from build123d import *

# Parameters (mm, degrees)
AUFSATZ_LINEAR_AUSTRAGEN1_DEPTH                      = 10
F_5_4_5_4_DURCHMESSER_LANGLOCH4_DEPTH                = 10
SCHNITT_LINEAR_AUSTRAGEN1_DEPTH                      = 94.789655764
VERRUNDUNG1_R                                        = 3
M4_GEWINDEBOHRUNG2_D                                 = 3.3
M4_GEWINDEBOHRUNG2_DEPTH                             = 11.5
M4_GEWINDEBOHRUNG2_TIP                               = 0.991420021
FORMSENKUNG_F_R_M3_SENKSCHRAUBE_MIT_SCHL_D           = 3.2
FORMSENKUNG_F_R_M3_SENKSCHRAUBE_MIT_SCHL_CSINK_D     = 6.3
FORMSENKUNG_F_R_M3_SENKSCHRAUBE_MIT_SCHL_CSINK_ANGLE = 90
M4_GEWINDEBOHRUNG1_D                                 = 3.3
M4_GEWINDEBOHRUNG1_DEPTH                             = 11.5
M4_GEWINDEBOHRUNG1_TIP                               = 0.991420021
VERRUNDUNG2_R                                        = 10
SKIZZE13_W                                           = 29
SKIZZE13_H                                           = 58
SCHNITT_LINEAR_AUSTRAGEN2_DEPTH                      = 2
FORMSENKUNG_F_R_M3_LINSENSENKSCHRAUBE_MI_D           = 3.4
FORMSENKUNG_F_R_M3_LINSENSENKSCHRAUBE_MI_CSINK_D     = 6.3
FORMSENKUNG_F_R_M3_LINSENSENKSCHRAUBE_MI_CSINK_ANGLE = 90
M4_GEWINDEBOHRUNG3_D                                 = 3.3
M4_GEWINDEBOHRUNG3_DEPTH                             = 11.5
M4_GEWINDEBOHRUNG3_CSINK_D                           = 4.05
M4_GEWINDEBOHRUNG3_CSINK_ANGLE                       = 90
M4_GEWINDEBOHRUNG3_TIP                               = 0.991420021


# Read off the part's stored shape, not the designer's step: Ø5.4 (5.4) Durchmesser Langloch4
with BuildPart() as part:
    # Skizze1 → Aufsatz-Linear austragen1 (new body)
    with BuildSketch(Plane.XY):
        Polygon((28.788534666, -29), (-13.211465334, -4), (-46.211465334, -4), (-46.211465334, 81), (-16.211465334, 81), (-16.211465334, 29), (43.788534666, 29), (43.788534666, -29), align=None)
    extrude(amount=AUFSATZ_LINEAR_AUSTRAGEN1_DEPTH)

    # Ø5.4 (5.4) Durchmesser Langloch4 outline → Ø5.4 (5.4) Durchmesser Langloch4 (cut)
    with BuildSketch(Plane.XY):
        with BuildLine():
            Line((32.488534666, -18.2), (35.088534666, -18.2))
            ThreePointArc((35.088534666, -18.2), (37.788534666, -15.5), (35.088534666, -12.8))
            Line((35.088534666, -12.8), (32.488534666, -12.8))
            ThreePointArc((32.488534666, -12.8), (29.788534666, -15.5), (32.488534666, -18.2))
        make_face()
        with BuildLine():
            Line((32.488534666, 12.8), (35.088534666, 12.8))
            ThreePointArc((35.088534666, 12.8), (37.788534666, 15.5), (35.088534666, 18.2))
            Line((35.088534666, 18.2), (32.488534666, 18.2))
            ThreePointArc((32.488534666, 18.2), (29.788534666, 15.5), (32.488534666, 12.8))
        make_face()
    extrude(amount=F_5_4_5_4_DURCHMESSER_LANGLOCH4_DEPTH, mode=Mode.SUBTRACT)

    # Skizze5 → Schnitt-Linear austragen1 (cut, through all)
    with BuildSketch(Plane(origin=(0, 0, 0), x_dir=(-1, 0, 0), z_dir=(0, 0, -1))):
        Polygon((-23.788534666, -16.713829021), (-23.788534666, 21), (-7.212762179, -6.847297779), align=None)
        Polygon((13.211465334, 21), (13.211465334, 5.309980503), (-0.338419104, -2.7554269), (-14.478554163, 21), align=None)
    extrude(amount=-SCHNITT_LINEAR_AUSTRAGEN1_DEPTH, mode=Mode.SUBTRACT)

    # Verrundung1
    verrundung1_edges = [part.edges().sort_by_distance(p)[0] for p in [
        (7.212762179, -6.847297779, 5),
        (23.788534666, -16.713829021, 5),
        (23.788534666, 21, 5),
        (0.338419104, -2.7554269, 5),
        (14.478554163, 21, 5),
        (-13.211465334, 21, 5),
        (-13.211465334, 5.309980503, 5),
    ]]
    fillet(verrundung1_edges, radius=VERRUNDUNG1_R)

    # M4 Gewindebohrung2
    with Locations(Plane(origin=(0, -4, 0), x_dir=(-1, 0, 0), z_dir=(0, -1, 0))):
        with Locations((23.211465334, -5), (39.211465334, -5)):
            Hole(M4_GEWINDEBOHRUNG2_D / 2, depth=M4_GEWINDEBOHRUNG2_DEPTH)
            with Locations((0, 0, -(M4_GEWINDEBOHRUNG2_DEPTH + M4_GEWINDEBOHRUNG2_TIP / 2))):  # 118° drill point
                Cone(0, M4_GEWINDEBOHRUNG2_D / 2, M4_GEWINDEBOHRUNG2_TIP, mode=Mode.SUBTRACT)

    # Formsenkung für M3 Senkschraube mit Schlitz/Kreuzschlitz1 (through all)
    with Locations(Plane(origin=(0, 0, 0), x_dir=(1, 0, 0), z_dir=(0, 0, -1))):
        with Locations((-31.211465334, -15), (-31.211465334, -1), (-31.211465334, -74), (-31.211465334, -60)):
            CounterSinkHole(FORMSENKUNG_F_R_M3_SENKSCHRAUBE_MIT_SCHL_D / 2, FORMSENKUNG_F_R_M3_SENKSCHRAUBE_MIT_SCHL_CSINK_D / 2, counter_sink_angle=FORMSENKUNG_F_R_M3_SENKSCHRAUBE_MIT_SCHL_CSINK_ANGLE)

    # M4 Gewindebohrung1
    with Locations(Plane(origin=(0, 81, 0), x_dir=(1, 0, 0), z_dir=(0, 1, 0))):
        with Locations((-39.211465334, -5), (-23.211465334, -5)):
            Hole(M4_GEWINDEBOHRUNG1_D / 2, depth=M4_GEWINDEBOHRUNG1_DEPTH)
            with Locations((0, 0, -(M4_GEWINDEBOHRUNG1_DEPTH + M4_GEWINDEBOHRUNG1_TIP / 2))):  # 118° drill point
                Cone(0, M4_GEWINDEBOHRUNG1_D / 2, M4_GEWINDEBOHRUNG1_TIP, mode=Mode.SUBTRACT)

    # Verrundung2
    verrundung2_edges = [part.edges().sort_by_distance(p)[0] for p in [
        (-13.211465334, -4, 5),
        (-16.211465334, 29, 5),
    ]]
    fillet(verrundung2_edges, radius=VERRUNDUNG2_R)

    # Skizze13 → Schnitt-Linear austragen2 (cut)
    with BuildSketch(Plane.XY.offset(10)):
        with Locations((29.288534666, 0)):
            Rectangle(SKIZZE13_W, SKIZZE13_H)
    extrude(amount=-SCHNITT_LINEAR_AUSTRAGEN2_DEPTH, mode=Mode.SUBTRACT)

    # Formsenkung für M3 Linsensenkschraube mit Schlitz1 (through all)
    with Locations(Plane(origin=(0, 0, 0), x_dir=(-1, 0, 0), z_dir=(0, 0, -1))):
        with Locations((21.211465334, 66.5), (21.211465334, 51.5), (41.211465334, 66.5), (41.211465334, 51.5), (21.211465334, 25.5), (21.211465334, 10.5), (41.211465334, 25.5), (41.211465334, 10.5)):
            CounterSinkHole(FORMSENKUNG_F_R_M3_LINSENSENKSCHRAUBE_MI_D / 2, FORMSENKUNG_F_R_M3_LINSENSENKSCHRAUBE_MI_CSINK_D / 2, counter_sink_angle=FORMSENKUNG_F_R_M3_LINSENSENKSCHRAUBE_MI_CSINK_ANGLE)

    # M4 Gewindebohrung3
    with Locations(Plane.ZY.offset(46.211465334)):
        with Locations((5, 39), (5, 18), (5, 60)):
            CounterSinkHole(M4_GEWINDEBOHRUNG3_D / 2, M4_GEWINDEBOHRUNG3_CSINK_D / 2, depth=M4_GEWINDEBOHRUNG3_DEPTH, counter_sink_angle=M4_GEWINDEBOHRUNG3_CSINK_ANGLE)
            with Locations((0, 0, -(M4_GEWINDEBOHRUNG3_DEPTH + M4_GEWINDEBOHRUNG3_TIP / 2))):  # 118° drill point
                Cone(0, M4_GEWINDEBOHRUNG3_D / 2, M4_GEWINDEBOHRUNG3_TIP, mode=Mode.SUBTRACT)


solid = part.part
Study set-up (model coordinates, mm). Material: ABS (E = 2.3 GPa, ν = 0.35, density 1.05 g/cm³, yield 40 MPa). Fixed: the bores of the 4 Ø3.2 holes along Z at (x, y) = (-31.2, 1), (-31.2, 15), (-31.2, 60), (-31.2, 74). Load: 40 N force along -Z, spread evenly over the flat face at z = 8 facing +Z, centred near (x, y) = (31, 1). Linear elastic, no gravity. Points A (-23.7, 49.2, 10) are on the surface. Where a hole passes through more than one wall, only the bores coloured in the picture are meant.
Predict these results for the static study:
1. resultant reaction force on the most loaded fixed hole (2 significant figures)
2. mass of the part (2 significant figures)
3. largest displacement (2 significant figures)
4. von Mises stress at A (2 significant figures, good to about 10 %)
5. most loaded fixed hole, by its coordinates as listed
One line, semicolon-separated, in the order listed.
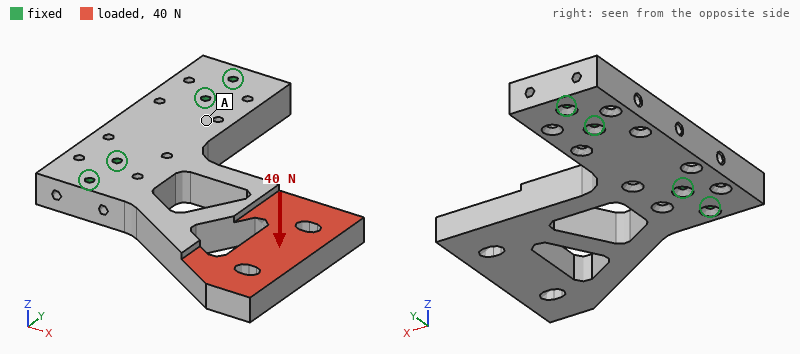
26 N; 44 g; 1.2 mm; 0.83 MPa; (-31.2, 15)
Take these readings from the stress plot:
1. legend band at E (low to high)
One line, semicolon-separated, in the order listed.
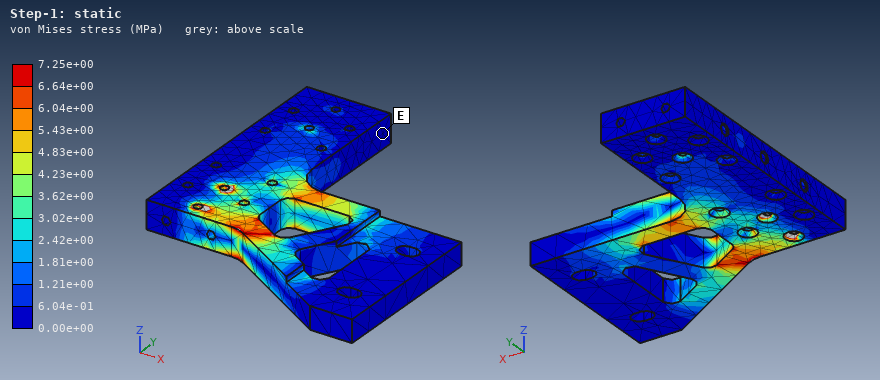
0.00e+00 to 6.04e-01 MPa
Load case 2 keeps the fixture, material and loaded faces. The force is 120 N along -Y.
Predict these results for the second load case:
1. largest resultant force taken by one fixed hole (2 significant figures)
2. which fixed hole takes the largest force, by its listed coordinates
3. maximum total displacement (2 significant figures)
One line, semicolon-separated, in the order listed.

230 N; (-31.2, 1); 0.54 mm
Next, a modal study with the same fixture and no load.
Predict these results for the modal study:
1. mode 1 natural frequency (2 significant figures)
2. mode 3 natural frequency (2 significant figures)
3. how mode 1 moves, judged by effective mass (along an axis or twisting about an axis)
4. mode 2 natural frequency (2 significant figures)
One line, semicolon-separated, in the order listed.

310 Hz; 770 Hz; along Z; 750 Hz
